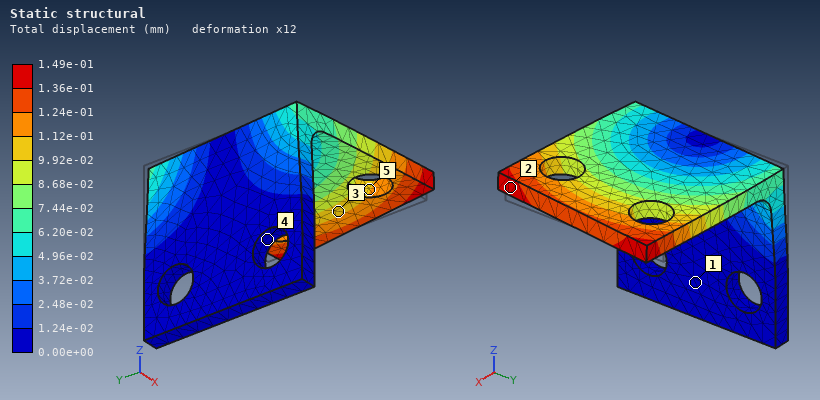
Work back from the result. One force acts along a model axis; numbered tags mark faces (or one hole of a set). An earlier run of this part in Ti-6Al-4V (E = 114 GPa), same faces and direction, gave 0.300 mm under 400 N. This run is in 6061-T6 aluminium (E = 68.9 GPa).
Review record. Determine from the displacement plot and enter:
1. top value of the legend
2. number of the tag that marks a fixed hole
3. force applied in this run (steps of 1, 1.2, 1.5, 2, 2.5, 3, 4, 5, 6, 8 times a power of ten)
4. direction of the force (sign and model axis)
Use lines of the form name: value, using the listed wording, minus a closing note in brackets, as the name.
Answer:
top value of the legend: 1.49e-01 mm
number of the tag that marks a fixed hole: 4
force applied in this run: 120 N
direction of the force: -Y
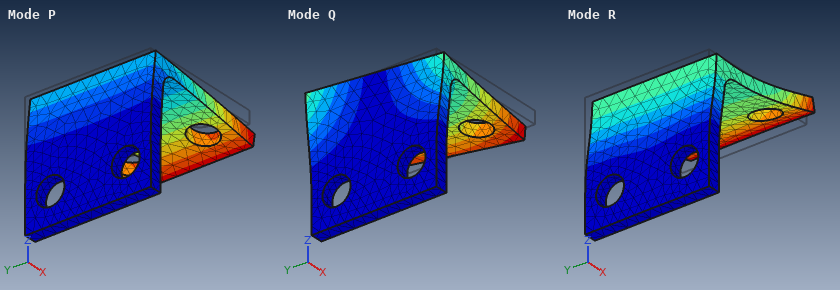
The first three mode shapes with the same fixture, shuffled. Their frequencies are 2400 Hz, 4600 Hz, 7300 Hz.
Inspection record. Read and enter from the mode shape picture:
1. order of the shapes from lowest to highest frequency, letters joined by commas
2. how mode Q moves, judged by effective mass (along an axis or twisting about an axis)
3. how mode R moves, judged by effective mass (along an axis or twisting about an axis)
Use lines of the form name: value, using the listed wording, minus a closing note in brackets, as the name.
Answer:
order of the shapes from lowest to highest frequency, letters joined by commas: P, Q, R
how mode Q moves, judged by effective mass: along Y
how mode R moves, judged by effective mass: along X
